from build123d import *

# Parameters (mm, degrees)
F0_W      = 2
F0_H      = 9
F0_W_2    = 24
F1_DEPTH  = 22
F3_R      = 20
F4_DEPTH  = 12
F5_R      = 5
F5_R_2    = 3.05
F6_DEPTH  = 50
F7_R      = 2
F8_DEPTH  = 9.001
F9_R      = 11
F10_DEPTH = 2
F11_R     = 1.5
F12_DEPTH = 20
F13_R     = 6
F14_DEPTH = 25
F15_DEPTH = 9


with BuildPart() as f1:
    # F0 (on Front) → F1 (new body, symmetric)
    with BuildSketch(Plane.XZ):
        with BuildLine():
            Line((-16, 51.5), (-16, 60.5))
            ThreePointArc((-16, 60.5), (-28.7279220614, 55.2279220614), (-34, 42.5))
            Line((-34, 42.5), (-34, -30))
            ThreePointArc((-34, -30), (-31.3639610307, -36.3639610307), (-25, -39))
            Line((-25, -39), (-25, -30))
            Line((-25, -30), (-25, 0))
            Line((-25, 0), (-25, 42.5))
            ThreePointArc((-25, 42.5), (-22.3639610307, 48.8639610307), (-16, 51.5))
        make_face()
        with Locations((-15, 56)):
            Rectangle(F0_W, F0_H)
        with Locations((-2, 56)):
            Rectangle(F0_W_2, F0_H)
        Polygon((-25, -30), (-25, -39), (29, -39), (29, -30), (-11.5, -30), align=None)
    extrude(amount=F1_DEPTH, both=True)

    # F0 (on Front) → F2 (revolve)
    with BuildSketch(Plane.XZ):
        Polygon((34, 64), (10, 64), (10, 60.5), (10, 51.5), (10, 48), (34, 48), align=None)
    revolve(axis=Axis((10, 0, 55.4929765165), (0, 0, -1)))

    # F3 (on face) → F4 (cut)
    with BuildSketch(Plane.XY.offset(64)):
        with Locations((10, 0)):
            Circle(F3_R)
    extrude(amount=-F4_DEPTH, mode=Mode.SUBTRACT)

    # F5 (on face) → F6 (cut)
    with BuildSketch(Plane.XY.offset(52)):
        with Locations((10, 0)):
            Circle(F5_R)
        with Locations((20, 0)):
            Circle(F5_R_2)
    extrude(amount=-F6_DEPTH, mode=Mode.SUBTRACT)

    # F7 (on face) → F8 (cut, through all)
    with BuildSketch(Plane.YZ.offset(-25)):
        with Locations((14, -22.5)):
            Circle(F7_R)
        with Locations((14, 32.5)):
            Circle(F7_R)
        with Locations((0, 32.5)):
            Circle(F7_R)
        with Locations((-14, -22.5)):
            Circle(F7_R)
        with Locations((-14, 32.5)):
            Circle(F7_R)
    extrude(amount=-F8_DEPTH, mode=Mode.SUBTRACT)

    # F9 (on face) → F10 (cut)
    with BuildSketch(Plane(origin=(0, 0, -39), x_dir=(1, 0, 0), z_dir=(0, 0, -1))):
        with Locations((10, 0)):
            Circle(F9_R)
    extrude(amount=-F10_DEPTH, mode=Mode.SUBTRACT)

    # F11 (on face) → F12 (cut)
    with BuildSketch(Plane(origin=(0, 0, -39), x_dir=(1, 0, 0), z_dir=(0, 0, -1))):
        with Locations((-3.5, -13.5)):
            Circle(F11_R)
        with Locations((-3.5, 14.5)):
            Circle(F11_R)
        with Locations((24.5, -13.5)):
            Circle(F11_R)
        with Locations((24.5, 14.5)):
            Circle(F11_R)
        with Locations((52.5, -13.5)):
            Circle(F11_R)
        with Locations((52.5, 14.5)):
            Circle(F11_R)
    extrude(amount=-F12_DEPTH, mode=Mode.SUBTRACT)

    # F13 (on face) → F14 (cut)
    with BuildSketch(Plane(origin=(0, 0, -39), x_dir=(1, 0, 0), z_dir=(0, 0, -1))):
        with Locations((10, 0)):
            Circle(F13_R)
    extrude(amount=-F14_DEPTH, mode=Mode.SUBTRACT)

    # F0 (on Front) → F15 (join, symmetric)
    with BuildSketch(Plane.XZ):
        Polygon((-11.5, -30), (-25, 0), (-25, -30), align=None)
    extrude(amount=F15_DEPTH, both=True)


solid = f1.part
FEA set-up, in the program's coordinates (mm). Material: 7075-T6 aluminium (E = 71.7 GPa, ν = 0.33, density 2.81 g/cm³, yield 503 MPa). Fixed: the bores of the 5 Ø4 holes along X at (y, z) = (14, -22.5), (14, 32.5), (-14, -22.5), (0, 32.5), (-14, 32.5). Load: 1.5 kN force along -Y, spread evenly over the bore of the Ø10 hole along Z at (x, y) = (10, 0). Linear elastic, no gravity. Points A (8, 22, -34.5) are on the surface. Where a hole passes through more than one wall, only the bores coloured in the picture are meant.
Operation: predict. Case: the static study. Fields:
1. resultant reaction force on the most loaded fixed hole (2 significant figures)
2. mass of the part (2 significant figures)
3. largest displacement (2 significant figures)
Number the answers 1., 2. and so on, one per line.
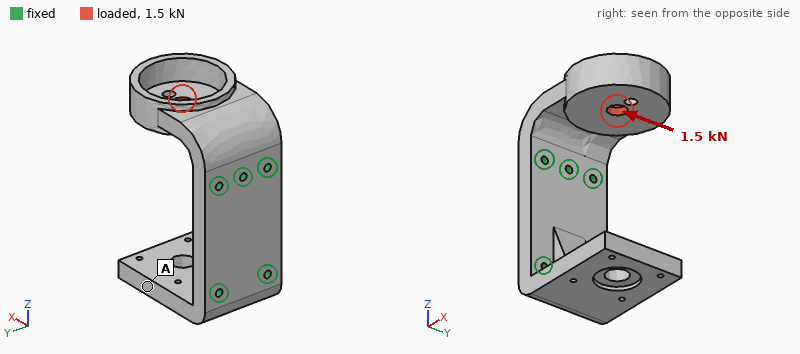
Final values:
1. 1.9 kN
2. 220 g
3. 0.18 mm
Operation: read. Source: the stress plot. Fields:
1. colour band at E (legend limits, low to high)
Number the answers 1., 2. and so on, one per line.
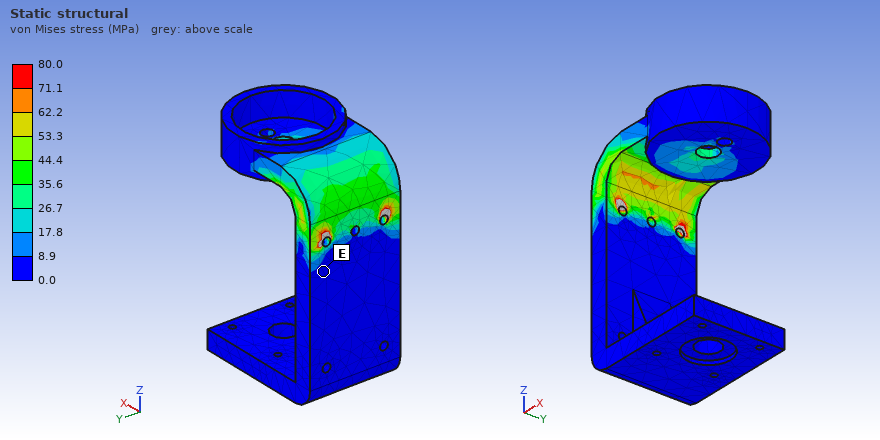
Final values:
1. 0.0 to 8.9 MPa
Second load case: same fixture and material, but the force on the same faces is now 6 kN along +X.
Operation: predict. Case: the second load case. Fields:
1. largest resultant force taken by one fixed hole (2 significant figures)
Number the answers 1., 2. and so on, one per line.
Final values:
1. 2.2 kN
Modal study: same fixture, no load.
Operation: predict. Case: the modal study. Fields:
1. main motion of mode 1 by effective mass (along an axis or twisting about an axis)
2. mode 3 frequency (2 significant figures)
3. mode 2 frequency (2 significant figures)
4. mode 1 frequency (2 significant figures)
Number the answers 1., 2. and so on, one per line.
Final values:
1. along Z
2. 2600 Hz
3. 2600 Hz
4. 1400 Hz
